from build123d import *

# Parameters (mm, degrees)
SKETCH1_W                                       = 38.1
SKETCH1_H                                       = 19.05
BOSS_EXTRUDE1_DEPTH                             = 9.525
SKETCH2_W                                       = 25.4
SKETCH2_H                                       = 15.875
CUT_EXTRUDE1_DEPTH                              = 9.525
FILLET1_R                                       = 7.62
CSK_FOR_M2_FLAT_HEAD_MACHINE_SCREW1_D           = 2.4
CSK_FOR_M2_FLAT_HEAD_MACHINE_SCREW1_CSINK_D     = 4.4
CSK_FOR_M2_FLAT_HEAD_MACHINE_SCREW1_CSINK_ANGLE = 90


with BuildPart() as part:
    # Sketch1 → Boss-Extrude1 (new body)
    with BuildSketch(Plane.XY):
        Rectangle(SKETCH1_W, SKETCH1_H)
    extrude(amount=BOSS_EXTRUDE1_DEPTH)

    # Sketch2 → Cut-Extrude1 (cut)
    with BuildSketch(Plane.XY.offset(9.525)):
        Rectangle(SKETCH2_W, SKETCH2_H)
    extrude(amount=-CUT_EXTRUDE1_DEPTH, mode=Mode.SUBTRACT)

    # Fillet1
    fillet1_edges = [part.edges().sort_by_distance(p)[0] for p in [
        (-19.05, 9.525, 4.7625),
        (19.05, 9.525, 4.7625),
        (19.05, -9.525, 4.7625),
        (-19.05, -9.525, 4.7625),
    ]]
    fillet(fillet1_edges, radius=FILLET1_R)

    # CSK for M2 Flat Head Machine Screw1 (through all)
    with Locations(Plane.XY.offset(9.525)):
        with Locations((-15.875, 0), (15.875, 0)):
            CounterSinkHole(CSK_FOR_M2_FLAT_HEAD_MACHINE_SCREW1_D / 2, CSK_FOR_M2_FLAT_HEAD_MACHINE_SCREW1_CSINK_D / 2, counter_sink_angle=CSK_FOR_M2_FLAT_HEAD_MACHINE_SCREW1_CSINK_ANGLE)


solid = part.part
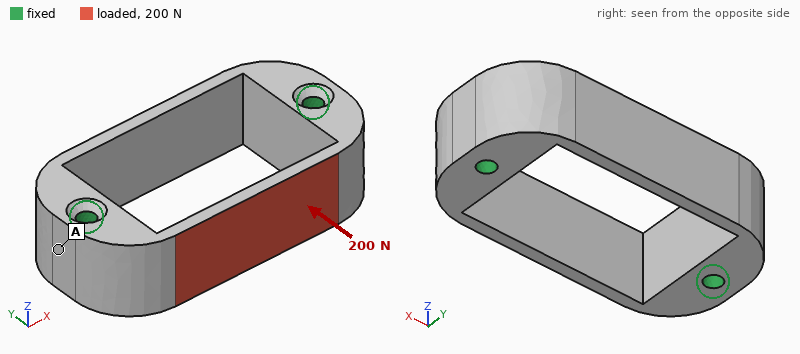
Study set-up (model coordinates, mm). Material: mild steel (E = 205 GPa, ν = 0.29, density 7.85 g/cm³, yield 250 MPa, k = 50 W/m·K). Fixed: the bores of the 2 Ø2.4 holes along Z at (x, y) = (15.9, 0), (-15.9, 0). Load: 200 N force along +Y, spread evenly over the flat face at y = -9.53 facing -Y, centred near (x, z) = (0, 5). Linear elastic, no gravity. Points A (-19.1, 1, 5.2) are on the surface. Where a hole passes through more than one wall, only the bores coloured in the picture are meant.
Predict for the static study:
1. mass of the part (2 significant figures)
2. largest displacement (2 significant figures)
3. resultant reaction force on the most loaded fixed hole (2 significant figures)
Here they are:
20 g
21 µm
140 N
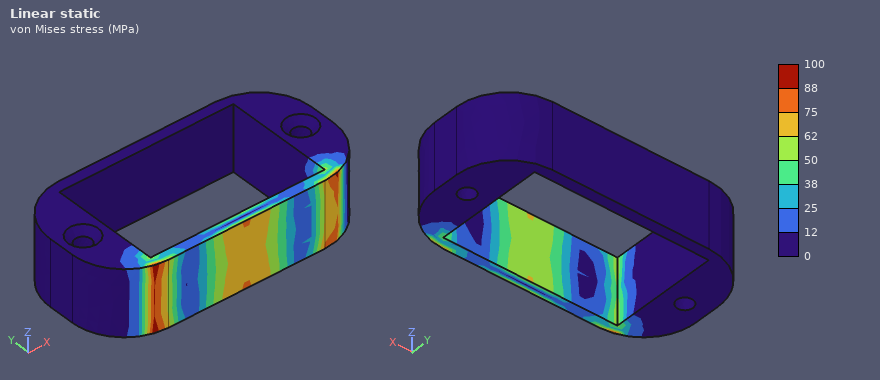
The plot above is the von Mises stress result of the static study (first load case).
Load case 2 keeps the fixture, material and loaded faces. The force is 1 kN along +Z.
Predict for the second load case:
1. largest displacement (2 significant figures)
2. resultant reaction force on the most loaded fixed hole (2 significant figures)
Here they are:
20 µm
500 N
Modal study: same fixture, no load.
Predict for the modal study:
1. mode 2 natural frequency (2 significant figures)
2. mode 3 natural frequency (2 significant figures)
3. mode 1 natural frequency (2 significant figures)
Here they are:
11 kHz
22 kHz
11 kHz
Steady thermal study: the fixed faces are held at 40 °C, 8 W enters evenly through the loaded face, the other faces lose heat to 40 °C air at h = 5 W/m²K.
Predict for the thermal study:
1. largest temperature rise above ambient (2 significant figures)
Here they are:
56 K
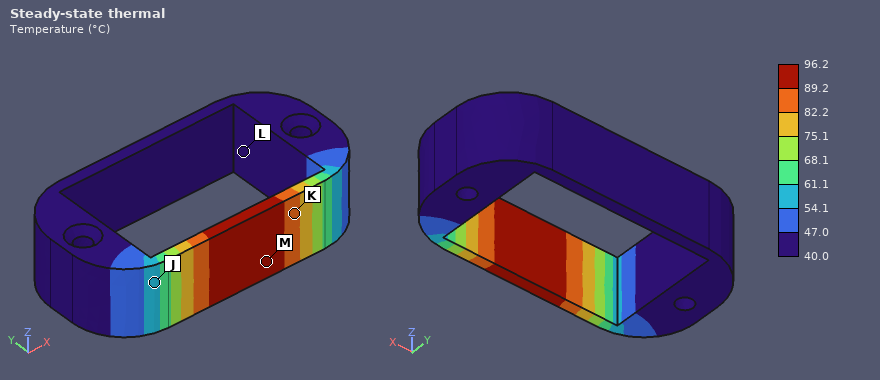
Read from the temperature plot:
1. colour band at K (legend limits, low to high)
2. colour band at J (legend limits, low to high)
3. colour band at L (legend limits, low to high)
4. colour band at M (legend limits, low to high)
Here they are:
82.2 to 89.2 °C
54.1 to 61.1 °C
40.0 to 47.0 °C
89.2 to 96.2 °C
